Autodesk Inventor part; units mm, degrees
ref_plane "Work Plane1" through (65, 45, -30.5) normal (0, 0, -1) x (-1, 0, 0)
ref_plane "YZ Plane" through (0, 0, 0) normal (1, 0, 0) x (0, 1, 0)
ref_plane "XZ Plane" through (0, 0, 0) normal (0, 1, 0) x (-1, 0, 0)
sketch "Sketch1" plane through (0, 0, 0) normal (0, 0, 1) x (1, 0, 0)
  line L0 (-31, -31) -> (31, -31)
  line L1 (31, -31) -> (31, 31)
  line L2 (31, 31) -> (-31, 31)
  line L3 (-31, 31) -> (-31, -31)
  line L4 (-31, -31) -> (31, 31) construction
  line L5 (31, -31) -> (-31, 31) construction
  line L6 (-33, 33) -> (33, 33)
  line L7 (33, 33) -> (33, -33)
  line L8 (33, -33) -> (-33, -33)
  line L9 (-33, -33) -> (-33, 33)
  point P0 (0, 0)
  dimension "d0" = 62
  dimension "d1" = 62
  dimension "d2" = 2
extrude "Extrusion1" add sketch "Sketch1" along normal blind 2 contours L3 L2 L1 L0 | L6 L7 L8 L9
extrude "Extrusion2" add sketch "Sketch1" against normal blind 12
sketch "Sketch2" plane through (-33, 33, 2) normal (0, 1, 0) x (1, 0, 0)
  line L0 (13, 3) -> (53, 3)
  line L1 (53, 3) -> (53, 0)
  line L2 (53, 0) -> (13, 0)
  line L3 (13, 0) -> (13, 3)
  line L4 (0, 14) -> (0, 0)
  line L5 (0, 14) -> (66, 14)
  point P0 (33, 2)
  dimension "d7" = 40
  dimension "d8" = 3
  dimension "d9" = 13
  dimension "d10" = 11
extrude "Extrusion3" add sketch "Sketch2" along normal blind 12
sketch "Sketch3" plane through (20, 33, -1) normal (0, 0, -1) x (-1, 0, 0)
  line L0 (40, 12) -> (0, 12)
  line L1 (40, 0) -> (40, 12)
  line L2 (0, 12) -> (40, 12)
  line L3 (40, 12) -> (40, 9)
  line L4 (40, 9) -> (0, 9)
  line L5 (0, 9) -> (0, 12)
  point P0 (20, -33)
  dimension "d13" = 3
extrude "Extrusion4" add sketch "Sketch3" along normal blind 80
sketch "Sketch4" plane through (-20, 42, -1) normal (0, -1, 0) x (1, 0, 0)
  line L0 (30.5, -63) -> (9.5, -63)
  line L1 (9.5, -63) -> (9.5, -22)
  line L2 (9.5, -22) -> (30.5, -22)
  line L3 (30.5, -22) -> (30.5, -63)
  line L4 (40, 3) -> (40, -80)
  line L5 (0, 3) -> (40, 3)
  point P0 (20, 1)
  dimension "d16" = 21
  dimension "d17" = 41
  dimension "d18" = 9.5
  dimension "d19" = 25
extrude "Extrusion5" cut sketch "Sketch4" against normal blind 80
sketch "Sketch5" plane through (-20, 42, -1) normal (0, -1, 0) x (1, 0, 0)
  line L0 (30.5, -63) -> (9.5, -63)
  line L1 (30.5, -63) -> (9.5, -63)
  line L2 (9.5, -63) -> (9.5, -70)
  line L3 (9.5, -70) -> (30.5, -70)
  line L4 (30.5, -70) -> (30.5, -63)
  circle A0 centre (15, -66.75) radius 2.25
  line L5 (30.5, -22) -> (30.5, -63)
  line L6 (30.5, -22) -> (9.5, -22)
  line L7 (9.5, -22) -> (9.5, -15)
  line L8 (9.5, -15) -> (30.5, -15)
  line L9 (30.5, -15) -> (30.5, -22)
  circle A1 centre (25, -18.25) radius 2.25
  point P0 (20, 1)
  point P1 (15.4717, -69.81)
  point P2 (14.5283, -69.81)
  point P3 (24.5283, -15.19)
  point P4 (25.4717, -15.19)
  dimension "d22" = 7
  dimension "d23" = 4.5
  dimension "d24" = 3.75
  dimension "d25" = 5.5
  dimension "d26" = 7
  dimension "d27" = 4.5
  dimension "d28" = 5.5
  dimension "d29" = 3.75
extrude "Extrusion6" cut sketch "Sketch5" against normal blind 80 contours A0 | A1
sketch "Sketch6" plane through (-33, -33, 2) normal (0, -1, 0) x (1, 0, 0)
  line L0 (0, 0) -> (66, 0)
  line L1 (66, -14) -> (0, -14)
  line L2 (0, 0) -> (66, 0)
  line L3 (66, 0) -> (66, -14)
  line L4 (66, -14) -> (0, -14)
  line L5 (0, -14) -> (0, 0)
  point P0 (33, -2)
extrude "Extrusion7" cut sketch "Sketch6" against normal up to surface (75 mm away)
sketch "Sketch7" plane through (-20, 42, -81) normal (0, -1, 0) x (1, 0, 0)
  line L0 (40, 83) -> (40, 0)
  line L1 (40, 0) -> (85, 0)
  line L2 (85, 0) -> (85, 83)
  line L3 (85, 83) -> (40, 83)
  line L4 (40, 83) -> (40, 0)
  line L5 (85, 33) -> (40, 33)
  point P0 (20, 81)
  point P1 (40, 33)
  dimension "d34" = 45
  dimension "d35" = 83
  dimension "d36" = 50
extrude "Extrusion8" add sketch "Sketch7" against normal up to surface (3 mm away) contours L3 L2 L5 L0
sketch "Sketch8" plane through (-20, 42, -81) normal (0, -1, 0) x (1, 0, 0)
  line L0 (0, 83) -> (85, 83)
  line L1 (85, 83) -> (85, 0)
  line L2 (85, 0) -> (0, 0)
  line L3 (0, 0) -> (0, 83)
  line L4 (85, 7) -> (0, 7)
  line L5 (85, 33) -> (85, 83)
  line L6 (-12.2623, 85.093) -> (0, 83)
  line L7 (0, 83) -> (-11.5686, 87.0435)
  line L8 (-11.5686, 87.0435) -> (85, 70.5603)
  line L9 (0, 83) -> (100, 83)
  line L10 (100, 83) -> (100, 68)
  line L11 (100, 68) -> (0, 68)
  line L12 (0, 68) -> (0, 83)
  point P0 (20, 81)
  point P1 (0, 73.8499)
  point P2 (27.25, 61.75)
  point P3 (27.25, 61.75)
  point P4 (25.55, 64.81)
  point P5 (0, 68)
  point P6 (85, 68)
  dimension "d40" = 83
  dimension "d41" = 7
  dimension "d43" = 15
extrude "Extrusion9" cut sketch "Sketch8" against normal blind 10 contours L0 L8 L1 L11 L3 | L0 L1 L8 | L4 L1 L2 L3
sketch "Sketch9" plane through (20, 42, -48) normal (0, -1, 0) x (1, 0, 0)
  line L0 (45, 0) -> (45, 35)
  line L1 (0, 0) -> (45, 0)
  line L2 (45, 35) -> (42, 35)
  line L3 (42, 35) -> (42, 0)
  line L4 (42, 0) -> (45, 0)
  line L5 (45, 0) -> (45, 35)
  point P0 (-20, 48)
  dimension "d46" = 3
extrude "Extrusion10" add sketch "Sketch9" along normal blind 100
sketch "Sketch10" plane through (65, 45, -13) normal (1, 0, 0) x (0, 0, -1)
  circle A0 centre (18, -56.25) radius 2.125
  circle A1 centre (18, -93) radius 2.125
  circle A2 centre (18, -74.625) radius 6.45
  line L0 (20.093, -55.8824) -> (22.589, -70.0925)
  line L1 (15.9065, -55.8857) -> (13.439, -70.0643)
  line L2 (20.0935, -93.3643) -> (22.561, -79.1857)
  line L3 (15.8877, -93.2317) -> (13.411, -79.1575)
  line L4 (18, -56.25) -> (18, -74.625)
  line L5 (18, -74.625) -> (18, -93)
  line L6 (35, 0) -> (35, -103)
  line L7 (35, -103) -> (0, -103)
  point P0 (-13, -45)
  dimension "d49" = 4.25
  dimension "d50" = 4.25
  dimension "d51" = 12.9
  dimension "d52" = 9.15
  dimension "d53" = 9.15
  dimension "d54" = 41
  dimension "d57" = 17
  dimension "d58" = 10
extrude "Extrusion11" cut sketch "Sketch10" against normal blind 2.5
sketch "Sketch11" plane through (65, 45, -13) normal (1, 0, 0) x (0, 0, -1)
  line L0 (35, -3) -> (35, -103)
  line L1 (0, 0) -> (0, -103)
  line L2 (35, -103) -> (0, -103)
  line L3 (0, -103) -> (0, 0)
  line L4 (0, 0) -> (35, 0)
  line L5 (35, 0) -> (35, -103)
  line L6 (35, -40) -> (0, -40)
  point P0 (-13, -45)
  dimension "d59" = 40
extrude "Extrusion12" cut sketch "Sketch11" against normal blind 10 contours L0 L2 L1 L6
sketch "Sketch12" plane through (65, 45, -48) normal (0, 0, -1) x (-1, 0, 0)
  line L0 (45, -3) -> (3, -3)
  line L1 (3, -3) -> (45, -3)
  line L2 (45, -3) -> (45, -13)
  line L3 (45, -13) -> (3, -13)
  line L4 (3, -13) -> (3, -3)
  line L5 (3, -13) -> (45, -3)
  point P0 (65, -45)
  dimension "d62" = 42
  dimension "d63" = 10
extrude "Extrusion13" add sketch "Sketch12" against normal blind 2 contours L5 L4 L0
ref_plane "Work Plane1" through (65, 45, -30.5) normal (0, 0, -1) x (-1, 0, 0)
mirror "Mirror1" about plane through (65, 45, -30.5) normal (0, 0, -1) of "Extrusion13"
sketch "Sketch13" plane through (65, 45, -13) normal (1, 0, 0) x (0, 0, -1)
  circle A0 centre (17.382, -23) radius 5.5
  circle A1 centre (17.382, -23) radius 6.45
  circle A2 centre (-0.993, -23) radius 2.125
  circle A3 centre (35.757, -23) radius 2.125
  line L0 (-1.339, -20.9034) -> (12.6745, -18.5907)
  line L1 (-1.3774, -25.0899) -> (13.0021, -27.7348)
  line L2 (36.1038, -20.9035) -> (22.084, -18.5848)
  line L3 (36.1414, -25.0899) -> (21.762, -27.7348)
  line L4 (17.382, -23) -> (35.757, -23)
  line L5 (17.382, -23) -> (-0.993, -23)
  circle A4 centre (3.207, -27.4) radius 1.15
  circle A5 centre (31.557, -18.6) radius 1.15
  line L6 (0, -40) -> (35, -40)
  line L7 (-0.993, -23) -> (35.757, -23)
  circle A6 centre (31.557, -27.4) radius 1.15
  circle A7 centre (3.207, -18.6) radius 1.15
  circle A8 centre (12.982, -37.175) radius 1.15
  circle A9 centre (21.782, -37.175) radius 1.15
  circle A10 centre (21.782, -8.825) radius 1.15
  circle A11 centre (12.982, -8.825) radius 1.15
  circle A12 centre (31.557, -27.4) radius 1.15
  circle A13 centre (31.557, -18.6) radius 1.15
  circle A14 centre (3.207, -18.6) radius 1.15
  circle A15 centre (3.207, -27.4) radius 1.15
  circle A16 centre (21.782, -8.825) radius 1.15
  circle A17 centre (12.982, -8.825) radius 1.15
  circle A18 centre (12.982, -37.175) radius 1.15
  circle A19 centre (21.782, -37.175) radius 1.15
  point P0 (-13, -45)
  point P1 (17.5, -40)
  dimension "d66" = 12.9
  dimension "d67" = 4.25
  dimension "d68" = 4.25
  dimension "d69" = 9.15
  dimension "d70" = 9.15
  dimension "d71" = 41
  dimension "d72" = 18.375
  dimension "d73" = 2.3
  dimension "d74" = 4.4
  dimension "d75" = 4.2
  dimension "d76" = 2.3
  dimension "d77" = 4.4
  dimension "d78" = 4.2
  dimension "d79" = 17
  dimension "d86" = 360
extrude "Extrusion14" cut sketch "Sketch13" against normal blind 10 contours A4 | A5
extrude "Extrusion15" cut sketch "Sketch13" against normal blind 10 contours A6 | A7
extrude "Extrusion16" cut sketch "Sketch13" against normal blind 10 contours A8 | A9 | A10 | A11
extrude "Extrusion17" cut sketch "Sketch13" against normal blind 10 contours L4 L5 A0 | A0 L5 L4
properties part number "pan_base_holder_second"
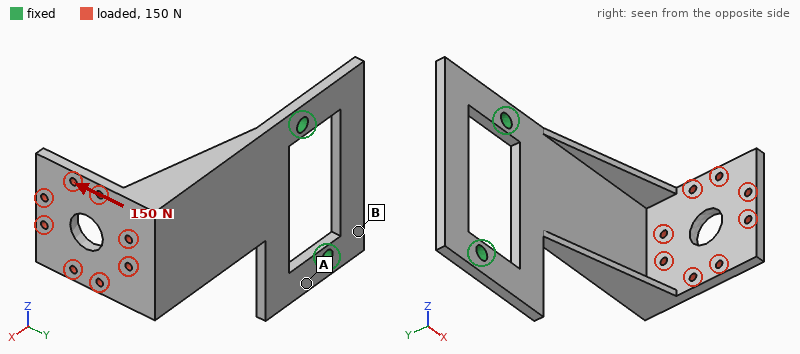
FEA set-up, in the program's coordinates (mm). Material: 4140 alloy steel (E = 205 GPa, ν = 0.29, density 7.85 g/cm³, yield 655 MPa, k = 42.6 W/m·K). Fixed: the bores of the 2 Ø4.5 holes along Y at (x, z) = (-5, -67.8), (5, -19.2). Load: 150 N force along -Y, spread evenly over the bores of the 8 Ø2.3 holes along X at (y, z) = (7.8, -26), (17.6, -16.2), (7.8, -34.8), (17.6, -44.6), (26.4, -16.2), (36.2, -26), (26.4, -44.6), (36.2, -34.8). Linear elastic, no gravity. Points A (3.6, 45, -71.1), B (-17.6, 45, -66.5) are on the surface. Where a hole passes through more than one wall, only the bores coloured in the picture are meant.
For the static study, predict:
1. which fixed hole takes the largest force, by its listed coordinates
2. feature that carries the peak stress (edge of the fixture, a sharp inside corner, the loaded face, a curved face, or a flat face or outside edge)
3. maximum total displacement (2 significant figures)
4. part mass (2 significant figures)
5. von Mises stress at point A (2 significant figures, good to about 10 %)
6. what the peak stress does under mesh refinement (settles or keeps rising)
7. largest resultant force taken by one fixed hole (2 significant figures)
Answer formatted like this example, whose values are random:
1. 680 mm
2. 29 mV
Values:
1. (5, -19.2)
2. edge of the fixture
3. 1.2 mm
4. 110 g
5. 130 MPa
6. keeps rising
7. 130 N
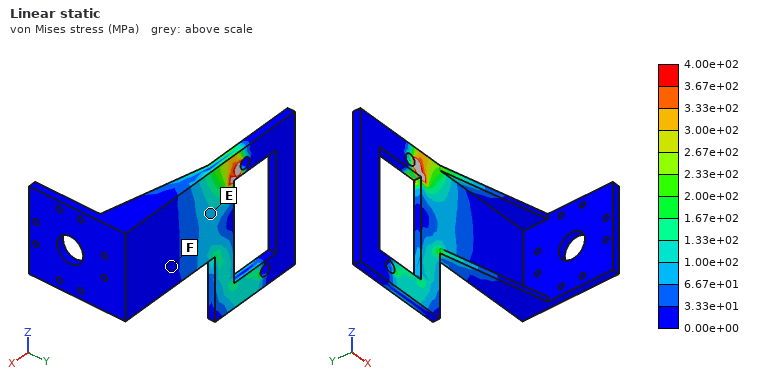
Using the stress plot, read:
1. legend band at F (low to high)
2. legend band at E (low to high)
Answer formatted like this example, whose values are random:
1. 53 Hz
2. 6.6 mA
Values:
1. 0.00e+00 to 3.33e+01 MPa
2. 6.67e+01 to 1.00e+02 MPa
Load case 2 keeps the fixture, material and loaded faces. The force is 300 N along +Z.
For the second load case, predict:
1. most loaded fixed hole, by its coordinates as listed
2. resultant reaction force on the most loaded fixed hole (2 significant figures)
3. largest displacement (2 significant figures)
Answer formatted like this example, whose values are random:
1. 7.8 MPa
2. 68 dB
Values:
1. (-5, -67.8)
2. 420 N
3. 0.54 mm
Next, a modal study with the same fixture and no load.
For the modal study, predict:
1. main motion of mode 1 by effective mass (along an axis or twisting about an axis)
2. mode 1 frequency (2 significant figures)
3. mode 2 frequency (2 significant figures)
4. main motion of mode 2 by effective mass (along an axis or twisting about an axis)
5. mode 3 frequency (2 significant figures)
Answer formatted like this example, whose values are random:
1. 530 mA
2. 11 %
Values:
1. along Y
2. 290 Hz
3. 830 Hz
4. along Z
5. 1800 Hz
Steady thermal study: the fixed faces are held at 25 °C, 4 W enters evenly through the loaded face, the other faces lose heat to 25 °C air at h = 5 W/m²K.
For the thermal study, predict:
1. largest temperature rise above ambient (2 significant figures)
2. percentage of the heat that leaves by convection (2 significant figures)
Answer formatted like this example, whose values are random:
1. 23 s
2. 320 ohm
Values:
1. 59 K
2. 37 %
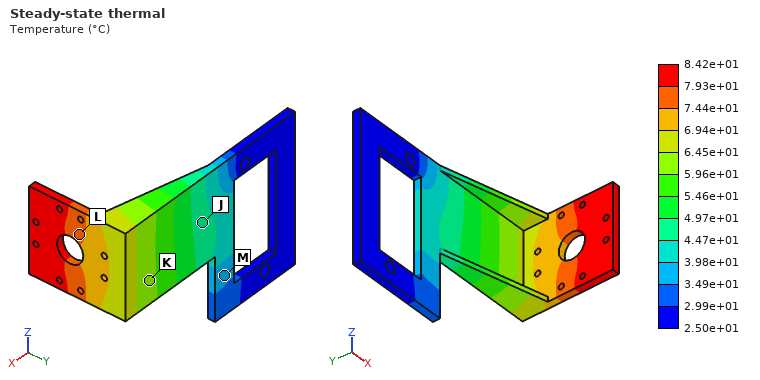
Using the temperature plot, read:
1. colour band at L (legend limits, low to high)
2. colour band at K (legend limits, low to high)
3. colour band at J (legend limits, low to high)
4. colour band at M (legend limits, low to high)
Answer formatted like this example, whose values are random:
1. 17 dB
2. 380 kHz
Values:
1. 7.44e+01 to 7.93e+01 °C
2. 5.96e+01 to 6.45e+01 °C
3. 4.47e+01 to 4.97e+01 °C
4. 3.49e+01 to 3.98e+01 °C
